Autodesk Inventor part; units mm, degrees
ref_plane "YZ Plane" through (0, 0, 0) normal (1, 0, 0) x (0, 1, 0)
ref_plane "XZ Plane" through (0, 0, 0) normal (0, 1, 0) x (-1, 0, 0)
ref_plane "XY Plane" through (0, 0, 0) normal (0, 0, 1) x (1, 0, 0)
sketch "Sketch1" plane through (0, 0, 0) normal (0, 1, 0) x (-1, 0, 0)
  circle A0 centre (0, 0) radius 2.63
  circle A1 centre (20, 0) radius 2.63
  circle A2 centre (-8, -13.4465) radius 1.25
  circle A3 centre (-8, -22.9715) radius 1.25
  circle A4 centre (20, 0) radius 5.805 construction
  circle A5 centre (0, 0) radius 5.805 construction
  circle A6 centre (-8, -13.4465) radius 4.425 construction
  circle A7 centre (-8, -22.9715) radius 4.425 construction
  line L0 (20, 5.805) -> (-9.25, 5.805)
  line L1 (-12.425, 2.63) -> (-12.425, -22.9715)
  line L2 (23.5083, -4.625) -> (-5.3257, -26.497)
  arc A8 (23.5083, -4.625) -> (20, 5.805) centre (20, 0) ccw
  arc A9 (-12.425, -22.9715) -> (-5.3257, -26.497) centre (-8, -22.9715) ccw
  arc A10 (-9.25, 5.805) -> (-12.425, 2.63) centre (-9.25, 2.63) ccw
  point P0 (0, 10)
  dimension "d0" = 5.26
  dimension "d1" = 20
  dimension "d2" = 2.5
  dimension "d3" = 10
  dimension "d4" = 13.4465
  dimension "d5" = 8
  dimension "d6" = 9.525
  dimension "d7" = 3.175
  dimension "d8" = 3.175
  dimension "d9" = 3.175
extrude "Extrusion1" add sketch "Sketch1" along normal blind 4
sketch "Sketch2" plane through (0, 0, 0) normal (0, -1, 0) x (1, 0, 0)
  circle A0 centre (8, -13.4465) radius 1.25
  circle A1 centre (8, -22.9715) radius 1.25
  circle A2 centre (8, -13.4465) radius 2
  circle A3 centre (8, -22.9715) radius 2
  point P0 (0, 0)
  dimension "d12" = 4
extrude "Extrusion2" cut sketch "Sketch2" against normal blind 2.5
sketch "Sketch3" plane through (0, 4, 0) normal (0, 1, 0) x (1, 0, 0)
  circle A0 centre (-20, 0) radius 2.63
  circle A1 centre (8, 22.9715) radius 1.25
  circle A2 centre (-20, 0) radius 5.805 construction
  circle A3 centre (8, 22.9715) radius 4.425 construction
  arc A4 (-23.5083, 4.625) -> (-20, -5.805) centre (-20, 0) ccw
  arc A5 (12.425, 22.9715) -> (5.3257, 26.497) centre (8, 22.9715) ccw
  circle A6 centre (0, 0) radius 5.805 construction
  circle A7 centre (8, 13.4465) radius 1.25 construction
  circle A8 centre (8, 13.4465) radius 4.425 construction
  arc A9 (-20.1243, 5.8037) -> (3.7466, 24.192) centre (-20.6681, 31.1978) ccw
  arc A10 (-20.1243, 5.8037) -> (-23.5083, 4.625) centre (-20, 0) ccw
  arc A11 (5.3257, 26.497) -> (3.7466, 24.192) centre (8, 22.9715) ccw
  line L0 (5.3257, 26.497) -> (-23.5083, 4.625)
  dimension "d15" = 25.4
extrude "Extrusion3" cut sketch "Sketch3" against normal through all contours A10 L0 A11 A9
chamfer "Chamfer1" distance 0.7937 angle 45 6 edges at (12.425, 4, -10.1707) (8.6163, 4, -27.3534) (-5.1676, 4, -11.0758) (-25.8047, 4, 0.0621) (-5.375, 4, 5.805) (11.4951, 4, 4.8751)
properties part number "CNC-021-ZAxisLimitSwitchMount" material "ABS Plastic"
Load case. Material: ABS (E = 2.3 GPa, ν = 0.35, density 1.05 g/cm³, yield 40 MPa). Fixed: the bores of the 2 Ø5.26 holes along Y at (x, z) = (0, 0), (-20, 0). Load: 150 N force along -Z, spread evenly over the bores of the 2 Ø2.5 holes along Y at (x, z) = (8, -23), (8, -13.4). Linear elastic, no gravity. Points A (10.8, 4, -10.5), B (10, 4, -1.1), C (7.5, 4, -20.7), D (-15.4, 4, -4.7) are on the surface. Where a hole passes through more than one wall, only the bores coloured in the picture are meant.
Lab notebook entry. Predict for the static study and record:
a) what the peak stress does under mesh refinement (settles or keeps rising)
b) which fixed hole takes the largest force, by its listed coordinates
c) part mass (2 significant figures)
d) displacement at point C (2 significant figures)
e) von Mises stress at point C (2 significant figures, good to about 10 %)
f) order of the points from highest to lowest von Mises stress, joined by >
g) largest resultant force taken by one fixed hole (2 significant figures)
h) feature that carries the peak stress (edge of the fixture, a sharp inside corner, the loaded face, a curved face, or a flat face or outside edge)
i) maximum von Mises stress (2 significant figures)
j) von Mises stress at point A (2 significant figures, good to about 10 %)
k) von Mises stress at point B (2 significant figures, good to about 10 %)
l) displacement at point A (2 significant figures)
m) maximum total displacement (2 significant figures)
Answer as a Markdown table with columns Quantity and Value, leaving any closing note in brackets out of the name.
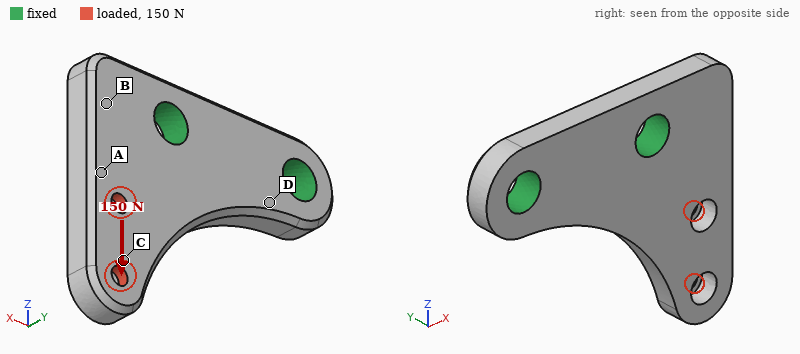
| Quantity | Value |
|---|---|
| what the peak stress does under mesh refinement | settles |
| which fixed hole takes the largest force, by its listed coordinates | (0, 0) |
| part mass | 2.7 g |
| displacement at point C | 0.21 mm |
| von Mises stress at point C | 7.0 MPa |
| order of the points from highest to lowest von Mises stress, joined by > | A > C > B > D |
| largest resultant force taken by one fixed hole | 180 N |
| feature that carries the peak stress | the loaded face |
| maximum von Mises stress | 23 MPa |
| von Mises stress at point A | 9.9 MPa |
| von Mises stress at point B | 3.9 MPa |
| displacement at point A | 0.093 mm |
| maximum total displacement | 0.34 mm |
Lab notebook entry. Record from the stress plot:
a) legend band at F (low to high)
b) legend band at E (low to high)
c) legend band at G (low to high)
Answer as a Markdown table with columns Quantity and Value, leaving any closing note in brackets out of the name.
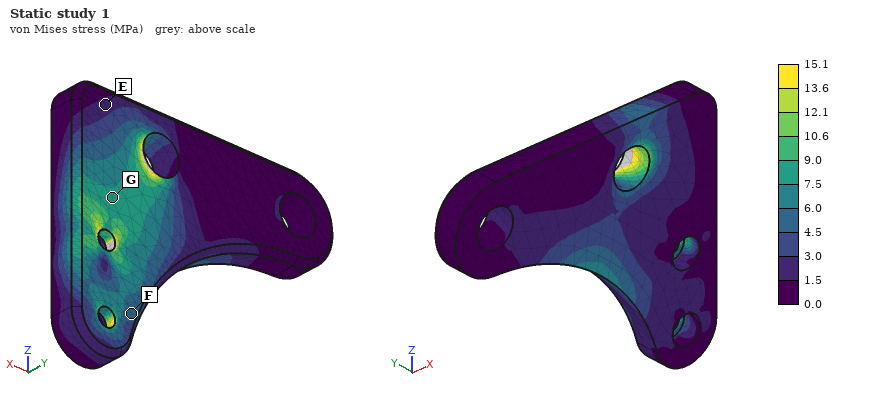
| Quantity | Value |
|---|---|
| legend band at F | 4.5 to 6.0 MPa |
| legend band at E | 1.5 to 3.0 MPa |
| legend band at G | 7.5 to 9.0 MPa |
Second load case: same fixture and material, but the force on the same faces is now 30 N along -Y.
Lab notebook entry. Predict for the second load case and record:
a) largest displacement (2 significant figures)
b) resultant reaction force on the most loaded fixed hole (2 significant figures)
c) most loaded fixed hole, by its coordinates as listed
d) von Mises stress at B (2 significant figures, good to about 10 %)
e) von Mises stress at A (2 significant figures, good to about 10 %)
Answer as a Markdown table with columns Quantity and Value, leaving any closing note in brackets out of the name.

| Quantity | Value |
|---|---|
| largest displacement | 0.57 mm |
| resultant reaction force on the most loaded fixed hole | 36 N |
| most loaded fixed hole, by its coordinates as listed | (0, 0) |
| von Mises stress at B | 5.0 MPa |
| von Mises stress at A | 5.8 MPa |
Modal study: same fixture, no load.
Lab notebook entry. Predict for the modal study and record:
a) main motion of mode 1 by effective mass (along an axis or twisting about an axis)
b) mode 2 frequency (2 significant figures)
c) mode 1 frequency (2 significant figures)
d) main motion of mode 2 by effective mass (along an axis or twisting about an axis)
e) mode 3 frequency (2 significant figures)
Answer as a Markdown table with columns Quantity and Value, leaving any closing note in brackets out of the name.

| Quantity | Value |
|---|---|
| main motion of mode 1 by effective mass | along Y |
| mode 2 frequency | 5200 Hz |
| mode 1 frequency | 1900 Hz |
| main motion of mode 2 by effective mass | along X |
| mode 3 frequency | 5800 Hz |
